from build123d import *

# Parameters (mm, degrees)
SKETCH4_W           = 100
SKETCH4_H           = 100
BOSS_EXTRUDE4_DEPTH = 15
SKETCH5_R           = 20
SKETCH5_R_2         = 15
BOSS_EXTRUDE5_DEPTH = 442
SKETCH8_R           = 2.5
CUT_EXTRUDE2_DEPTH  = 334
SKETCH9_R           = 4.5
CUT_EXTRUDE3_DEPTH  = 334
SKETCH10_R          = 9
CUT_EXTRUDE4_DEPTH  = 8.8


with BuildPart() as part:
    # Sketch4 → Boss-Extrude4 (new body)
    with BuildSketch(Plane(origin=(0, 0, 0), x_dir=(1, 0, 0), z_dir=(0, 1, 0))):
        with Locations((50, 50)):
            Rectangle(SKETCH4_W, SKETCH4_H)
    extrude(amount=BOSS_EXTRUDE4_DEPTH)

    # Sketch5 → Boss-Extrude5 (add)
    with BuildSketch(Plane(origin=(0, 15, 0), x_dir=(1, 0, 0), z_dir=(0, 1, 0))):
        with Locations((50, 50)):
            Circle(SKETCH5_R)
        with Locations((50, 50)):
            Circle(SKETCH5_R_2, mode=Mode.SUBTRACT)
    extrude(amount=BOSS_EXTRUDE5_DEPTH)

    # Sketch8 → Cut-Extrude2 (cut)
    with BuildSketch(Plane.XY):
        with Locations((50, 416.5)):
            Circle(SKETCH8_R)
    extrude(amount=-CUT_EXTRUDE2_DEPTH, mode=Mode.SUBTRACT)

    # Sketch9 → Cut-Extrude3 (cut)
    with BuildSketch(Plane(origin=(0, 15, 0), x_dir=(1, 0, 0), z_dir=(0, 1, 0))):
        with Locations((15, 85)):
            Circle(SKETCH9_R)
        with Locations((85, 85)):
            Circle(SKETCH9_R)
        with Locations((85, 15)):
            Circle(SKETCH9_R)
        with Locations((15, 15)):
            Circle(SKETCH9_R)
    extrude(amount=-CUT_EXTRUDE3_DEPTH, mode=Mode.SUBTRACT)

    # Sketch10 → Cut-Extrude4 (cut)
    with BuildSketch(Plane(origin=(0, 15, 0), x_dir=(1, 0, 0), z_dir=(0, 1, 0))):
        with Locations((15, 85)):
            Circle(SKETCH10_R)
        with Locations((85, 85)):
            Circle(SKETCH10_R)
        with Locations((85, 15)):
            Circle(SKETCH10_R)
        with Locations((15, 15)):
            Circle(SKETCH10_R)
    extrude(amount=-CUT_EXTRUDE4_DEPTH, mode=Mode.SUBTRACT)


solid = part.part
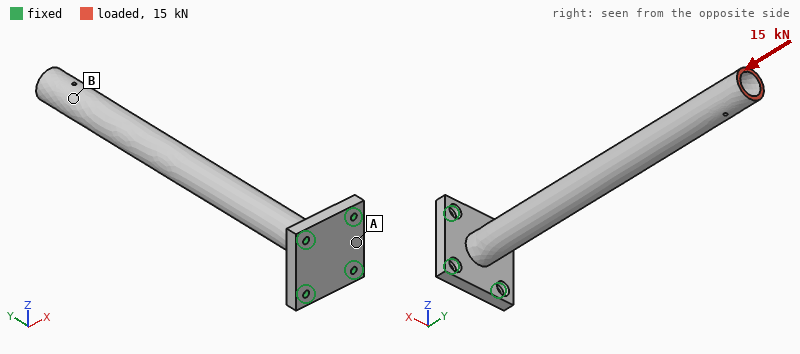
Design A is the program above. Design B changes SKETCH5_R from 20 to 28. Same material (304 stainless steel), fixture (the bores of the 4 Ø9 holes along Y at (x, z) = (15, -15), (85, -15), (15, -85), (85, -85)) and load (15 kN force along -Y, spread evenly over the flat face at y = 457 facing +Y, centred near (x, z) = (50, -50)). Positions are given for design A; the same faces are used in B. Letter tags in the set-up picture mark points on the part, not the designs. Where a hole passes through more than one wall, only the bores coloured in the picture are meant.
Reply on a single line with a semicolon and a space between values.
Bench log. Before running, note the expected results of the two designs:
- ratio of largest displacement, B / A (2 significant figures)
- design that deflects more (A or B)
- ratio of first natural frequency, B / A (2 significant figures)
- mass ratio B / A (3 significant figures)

0.37; A; 1.1; 2.39
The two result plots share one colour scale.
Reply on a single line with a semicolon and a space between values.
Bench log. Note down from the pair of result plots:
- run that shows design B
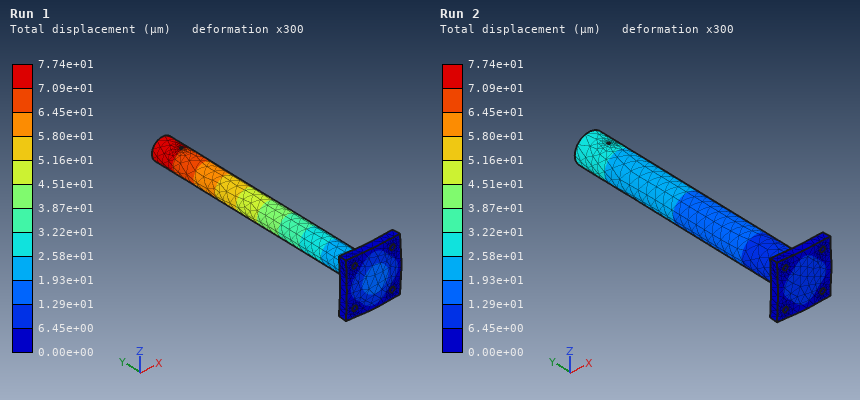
Run 2
